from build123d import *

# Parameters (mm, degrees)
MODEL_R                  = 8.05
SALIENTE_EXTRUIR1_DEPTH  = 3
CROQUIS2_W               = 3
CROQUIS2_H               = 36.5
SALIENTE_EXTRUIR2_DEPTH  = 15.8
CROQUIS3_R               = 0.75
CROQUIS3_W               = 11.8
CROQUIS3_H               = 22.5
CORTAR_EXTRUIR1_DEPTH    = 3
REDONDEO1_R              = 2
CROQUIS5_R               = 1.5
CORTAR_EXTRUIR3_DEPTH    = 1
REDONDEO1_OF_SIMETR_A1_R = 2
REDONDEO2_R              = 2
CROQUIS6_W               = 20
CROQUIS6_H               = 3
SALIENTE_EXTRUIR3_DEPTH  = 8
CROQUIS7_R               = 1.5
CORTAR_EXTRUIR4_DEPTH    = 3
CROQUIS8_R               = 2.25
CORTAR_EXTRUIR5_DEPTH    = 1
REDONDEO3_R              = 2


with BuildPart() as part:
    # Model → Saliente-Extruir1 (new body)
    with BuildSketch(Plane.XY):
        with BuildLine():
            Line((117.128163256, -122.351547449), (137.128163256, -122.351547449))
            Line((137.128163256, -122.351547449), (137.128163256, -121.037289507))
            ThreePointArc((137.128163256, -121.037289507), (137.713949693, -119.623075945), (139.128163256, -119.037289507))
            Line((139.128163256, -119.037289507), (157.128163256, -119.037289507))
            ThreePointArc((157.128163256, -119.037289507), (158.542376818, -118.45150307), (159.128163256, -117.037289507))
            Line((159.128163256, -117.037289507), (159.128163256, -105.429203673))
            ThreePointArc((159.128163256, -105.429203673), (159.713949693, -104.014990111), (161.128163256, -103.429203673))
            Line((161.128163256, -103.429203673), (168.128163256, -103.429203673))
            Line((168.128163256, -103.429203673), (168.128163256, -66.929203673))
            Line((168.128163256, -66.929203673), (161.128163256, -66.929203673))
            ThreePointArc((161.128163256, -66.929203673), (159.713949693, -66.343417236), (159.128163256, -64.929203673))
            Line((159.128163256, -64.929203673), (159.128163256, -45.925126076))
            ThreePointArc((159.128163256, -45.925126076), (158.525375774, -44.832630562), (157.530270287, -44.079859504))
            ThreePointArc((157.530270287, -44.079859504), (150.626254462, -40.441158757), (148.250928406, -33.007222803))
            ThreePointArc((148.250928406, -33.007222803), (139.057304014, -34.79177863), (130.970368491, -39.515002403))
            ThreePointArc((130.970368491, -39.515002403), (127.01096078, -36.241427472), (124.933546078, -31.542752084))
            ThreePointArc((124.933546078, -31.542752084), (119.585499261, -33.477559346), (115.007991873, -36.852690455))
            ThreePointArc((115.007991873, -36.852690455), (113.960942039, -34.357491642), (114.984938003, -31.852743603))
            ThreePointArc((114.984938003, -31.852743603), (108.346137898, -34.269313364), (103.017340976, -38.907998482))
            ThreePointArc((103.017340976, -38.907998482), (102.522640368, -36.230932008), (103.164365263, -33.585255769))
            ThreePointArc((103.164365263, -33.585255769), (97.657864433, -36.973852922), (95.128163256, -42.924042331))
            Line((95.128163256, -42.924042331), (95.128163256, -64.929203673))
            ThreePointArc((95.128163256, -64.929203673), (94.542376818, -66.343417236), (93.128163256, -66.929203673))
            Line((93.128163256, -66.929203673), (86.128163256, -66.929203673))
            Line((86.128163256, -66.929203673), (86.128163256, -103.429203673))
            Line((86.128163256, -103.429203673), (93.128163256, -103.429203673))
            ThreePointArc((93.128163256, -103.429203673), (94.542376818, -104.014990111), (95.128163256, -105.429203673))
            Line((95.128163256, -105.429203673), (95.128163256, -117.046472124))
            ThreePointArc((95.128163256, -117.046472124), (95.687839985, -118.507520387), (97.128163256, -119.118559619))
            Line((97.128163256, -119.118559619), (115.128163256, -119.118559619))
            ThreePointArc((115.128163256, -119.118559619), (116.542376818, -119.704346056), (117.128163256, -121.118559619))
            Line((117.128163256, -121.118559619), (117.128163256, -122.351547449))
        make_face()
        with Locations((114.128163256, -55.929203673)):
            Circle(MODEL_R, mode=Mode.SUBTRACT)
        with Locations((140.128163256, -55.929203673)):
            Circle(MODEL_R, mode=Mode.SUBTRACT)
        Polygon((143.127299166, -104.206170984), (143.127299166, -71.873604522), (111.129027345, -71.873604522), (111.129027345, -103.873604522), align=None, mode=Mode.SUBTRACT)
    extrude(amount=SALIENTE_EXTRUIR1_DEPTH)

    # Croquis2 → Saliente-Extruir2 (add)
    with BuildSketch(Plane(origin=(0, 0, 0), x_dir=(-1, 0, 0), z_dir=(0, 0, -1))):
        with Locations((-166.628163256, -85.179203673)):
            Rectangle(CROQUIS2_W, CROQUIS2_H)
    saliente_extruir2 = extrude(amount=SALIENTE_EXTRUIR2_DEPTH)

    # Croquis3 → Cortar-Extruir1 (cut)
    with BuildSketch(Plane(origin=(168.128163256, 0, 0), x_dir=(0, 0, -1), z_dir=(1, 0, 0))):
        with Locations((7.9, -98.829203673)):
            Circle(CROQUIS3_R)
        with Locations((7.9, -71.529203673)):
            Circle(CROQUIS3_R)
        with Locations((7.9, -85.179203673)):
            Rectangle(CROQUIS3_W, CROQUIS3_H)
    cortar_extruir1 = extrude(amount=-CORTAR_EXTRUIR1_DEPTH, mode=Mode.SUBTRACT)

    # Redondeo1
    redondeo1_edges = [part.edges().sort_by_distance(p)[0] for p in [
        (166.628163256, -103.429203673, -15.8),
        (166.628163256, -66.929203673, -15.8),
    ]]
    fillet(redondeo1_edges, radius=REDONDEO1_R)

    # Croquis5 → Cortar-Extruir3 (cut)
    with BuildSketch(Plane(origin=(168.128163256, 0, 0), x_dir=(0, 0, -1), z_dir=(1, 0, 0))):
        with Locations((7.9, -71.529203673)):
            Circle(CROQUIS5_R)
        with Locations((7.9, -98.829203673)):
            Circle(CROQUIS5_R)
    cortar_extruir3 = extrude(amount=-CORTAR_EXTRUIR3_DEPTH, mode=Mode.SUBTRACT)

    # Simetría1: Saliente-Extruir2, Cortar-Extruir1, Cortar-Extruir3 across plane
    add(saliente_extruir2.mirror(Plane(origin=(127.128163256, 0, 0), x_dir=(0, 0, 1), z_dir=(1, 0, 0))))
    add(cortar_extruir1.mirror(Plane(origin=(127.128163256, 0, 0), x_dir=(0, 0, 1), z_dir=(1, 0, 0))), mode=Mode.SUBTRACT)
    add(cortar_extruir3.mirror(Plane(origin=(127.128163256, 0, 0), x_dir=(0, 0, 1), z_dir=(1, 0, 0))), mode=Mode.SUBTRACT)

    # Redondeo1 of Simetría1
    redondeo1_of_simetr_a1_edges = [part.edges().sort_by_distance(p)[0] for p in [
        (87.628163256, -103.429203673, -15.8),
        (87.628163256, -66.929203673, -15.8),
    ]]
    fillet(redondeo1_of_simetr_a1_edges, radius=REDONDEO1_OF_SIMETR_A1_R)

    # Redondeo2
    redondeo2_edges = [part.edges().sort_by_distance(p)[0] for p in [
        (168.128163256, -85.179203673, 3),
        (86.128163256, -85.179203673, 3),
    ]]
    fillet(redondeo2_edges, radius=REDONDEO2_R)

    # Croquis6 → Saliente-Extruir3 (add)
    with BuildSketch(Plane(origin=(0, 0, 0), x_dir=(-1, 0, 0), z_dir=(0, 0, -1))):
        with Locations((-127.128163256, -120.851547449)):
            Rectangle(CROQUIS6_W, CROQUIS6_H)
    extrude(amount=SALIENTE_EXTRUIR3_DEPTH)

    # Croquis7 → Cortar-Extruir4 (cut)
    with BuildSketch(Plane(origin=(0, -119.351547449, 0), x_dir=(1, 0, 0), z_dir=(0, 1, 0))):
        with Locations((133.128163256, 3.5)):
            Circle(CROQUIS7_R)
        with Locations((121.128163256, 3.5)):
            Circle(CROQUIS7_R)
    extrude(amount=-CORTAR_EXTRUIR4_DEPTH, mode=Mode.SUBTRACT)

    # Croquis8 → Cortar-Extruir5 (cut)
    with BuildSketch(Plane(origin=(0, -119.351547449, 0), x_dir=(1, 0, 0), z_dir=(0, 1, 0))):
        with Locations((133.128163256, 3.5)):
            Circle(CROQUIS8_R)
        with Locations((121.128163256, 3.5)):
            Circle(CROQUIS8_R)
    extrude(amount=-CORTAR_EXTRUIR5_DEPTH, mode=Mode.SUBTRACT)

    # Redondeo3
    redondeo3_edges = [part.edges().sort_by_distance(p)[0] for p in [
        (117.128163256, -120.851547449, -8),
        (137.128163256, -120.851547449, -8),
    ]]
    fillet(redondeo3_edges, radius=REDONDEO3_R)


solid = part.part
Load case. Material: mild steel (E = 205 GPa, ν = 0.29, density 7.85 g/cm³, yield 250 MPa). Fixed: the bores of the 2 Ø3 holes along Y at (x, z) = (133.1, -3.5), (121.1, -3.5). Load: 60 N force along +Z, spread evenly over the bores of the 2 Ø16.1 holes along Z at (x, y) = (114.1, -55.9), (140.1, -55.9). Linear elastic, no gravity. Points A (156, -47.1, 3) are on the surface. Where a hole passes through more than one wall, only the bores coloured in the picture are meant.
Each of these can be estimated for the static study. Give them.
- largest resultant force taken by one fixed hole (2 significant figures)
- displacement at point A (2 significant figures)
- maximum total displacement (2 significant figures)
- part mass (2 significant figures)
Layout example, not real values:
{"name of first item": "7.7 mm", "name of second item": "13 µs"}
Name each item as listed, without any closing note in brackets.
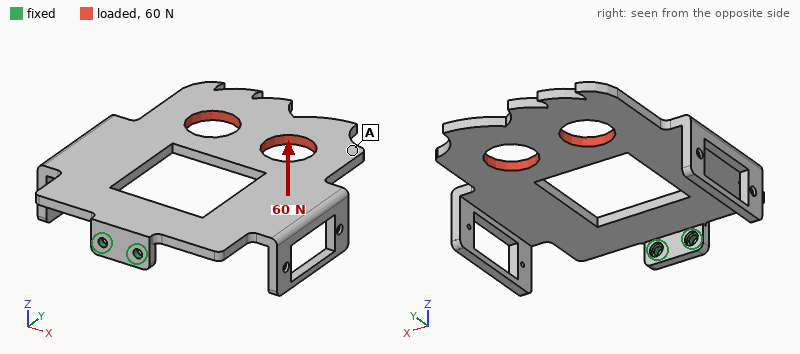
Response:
{"largest resultant force taken by one fixed hole": "61 N", "displacement at point A": "0.63 mm", "maximum total displacement": "0.80 mm", "part mass": "120 g"}
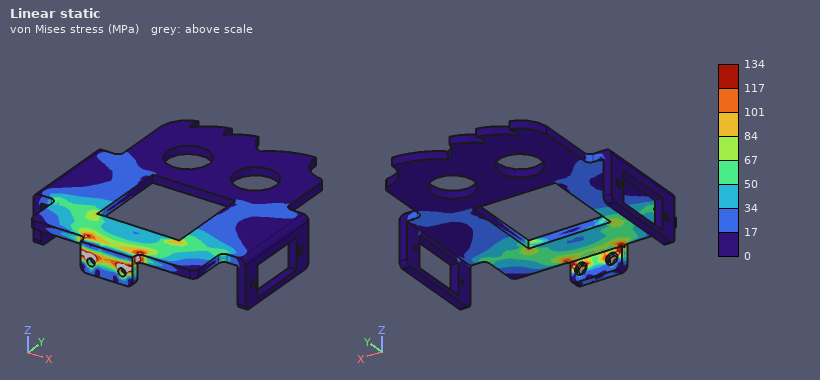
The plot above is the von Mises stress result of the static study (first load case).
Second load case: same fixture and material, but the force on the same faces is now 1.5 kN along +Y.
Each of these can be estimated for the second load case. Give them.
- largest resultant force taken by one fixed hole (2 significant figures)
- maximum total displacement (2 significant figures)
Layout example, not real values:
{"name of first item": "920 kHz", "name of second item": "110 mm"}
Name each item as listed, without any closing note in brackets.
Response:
{"largest resultant force taken by one fixed hole": "760 N", "maximum total displacement": "0.26 mm"}
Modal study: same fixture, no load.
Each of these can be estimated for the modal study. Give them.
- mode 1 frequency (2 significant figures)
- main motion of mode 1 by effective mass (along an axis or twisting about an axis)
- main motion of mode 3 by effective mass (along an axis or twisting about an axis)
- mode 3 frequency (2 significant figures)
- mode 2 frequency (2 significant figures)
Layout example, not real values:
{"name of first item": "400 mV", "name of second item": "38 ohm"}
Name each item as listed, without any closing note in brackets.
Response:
{"mode 1 frequency": "210 Hz", "main motion of mode 1 by effective mass": "along Z", "main motion of mode 3 by effective mass": "along X", "mode 3 frequency": "780 Hz", "mode 2 frequency": "470 Hz"}
